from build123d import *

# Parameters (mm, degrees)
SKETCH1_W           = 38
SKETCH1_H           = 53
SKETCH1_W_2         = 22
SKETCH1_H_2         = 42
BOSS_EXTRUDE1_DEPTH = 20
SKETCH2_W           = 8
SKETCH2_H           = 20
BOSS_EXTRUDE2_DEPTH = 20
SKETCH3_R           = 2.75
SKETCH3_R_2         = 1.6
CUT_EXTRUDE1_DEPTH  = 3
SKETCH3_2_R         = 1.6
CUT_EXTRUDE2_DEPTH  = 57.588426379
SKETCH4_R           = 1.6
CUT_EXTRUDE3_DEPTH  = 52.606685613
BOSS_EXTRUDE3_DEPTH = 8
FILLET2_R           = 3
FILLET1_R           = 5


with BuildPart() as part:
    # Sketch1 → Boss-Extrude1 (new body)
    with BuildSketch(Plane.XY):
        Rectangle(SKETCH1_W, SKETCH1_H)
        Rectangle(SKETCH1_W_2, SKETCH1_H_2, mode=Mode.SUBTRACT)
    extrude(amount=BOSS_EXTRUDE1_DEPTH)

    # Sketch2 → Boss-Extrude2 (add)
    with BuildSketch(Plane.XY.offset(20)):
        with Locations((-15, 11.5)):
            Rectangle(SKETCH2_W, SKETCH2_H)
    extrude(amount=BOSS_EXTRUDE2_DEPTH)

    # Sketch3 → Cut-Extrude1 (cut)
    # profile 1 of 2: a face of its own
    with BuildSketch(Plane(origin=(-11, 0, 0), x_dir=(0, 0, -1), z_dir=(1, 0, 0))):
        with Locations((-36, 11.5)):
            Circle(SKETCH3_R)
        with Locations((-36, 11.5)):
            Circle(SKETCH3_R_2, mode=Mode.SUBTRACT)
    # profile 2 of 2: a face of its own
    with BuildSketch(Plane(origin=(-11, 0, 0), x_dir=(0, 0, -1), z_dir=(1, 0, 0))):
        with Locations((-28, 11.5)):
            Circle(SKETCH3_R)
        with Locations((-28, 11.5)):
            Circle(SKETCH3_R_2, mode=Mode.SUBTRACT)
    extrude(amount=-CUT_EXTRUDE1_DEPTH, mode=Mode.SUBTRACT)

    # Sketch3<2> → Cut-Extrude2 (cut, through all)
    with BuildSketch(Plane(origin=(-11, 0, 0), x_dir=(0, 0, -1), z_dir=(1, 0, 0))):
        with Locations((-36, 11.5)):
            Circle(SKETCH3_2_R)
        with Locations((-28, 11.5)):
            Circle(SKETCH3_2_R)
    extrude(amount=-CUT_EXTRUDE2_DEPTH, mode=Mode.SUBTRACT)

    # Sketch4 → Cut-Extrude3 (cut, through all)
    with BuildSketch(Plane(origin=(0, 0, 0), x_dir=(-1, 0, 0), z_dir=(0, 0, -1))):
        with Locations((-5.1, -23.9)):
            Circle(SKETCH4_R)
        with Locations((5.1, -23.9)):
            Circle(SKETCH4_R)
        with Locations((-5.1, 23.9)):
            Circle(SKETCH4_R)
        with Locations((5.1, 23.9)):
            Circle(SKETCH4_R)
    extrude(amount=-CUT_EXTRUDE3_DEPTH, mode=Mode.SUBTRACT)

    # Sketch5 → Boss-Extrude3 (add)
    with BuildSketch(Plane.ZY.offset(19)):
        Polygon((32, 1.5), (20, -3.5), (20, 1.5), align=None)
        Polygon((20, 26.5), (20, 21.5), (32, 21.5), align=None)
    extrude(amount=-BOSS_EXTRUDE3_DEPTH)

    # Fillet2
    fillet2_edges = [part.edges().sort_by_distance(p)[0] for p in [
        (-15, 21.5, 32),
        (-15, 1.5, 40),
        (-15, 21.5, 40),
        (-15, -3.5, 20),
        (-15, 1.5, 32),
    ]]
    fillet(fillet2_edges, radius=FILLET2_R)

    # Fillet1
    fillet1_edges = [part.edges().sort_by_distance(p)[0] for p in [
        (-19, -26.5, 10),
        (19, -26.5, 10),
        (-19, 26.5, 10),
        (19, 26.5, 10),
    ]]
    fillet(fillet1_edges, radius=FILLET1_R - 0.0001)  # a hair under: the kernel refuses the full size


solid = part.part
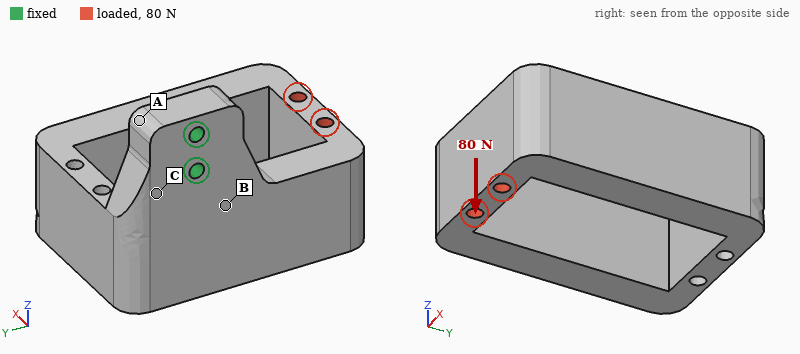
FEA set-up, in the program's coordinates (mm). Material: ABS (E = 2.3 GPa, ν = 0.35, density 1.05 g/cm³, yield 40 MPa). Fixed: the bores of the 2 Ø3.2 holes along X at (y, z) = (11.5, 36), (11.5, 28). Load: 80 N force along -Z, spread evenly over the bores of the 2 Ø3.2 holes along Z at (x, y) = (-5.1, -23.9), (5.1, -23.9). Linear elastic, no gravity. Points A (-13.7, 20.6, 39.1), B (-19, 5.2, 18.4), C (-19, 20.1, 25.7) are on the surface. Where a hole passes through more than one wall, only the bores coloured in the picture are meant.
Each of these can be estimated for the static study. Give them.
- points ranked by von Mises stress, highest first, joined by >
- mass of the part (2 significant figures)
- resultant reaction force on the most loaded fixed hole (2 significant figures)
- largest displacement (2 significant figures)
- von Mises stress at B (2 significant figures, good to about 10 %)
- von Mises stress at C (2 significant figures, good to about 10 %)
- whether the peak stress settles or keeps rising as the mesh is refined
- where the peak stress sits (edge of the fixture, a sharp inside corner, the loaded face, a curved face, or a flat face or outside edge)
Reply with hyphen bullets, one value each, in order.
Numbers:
- C > B > A
- 25 g
- 280 N
- 0.90 mm
- 3.5 MPa
- 6.5 MPa
- keeps rising
- edge of the fixture
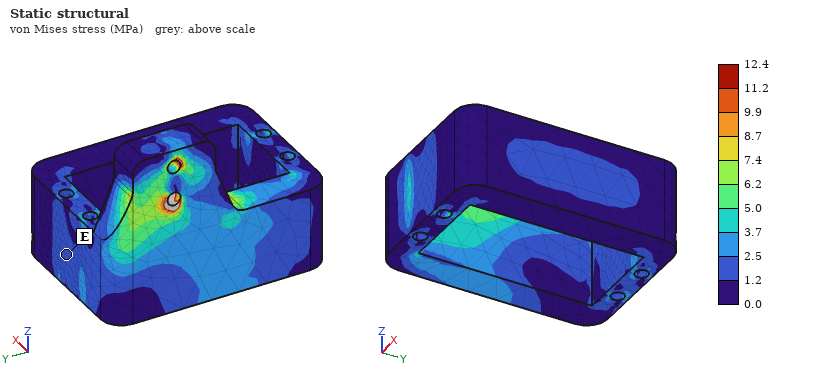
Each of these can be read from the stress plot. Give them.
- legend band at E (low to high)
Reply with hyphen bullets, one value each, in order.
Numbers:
- 1.2 to 2.5 MPa
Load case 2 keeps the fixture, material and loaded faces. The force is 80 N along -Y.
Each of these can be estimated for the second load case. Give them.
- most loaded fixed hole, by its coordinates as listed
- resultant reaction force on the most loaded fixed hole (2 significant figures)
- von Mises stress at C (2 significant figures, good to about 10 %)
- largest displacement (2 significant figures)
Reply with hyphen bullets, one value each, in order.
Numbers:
- (11.5, 28)
- 200 N
- 2.8 MPa
- 0.72 mm
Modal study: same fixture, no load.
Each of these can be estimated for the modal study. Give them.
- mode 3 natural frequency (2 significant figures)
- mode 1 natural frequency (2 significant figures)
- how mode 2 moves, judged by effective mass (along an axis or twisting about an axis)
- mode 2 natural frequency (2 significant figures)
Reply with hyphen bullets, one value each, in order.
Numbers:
- 960 Hz
- 360 Hz
- along Z
- 430 Hz
